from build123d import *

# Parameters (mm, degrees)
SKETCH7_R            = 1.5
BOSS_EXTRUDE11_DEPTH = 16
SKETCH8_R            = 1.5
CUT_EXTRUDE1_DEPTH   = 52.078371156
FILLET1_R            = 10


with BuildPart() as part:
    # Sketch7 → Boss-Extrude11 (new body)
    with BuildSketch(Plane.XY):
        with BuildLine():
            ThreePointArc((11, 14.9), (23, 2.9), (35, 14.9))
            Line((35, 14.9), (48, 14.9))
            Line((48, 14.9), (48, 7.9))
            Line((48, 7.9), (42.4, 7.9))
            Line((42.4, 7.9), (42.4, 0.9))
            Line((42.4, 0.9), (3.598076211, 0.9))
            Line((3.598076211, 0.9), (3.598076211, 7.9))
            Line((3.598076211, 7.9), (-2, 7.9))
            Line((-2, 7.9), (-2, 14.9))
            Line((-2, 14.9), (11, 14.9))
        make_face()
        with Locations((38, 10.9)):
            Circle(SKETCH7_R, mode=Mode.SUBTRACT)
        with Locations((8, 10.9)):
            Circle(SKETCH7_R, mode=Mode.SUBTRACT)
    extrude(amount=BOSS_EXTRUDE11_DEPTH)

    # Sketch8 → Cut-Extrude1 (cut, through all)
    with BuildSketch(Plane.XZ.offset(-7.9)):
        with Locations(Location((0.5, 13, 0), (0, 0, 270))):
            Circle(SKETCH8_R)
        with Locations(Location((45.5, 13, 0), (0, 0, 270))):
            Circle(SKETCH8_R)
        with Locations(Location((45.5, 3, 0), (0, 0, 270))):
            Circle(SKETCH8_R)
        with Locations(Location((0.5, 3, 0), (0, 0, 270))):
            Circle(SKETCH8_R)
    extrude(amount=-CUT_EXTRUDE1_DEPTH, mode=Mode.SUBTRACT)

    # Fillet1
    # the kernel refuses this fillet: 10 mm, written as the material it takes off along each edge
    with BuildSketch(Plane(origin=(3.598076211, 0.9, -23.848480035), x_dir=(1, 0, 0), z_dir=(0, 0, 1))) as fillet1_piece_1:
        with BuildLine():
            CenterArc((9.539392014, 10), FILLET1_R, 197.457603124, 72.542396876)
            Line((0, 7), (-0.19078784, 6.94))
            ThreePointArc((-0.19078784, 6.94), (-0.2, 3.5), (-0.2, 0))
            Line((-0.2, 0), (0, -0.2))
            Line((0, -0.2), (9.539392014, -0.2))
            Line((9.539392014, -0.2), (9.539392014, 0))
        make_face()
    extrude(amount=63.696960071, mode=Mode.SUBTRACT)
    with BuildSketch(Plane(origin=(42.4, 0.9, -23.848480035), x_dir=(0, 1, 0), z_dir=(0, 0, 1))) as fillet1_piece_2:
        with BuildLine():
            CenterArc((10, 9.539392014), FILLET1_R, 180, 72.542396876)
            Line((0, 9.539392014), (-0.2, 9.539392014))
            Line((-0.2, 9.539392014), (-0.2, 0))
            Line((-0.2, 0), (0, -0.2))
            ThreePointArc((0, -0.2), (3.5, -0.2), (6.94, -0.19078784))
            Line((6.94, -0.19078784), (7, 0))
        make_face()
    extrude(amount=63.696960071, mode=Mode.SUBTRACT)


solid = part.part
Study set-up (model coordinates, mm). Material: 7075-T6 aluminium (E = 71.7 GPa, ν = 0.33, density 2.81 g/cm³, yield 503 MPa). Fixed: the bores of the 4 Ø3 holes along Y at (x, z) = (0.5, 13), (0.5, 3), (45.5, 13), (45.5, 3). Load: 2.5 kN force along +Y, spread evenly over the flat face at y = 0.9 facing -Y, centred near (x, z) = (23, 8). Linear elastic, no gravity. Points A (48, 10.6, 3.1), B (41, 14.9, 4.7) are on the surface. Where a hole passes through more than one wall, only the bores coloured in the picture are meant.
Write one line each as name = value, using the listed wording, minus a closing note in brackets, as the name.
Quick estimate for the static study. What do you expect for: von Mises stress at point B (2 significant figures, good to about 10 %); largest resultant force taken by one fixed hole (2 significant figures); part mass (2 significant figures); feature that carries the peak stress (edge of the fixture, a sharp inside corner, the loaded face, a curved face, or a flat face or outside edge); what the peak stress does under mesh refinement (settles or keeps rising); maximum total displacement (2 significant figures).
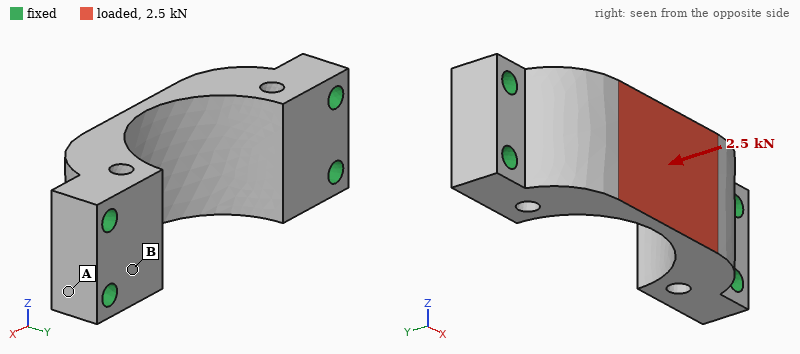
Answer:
von Mises stress at point B = 28 MPa
largest resultant force taken by one fixed hole = 1.1 kN
part mass = 15 g
feature that carries the peak stress = edge of the fixture
what the peak stress does under mesh refinement = keeps rising
maximum total displacement = 28 µm
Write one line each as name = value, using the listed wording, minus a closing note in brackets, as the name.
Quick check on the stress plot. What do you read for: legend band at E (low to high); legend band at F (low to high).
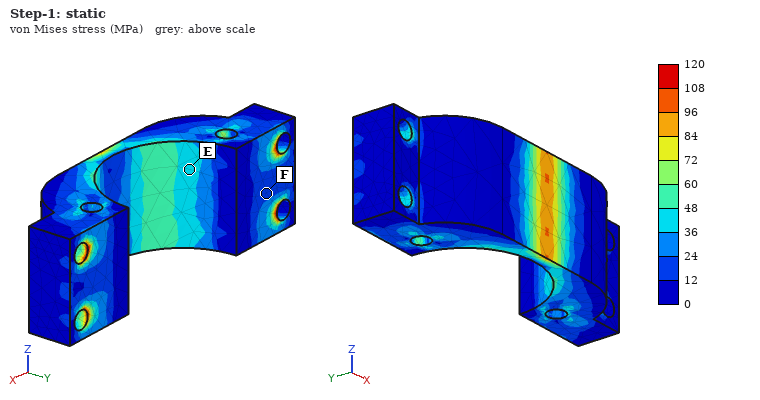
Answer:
legend band at E = 36 to 48 MPa
legend band at F = 12 to 24 MPa
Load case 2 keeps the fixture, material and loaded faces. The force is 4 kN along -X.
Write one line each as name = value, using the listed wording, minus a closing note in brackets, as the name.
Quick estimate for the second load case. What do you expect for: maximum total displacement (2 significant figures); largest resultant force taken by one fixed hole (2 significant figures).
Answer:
maximum total displacement = 23 µm
largest resultant force taken by one fixed hole = 1.1 kN
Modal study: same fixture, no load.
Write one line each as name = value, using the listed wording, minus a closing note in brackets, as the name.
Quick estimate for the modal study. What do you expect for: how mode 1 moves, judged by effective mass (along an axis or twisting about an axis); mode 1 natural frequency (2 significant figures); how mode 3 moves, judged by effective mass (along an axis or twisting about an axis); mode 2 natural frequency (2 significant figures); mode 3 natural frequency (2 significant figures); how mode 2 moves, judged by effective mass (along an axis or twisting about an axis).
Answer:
how mode 1 moves, judged by effective mass = along X
mode 1 natural frequency = 22 kHz
how mode 3 moves, judged by effective mass = along Y
mode 2 natural frequency = 23 kHz
mode 3 natural frequency = 27 kHz
how mode 2 moves, judged by effective mass = along Z
